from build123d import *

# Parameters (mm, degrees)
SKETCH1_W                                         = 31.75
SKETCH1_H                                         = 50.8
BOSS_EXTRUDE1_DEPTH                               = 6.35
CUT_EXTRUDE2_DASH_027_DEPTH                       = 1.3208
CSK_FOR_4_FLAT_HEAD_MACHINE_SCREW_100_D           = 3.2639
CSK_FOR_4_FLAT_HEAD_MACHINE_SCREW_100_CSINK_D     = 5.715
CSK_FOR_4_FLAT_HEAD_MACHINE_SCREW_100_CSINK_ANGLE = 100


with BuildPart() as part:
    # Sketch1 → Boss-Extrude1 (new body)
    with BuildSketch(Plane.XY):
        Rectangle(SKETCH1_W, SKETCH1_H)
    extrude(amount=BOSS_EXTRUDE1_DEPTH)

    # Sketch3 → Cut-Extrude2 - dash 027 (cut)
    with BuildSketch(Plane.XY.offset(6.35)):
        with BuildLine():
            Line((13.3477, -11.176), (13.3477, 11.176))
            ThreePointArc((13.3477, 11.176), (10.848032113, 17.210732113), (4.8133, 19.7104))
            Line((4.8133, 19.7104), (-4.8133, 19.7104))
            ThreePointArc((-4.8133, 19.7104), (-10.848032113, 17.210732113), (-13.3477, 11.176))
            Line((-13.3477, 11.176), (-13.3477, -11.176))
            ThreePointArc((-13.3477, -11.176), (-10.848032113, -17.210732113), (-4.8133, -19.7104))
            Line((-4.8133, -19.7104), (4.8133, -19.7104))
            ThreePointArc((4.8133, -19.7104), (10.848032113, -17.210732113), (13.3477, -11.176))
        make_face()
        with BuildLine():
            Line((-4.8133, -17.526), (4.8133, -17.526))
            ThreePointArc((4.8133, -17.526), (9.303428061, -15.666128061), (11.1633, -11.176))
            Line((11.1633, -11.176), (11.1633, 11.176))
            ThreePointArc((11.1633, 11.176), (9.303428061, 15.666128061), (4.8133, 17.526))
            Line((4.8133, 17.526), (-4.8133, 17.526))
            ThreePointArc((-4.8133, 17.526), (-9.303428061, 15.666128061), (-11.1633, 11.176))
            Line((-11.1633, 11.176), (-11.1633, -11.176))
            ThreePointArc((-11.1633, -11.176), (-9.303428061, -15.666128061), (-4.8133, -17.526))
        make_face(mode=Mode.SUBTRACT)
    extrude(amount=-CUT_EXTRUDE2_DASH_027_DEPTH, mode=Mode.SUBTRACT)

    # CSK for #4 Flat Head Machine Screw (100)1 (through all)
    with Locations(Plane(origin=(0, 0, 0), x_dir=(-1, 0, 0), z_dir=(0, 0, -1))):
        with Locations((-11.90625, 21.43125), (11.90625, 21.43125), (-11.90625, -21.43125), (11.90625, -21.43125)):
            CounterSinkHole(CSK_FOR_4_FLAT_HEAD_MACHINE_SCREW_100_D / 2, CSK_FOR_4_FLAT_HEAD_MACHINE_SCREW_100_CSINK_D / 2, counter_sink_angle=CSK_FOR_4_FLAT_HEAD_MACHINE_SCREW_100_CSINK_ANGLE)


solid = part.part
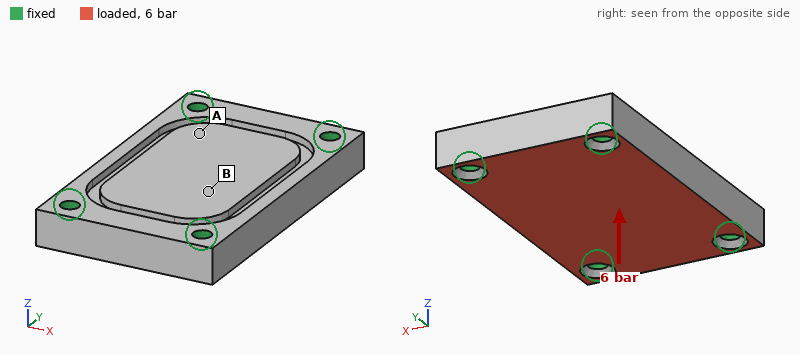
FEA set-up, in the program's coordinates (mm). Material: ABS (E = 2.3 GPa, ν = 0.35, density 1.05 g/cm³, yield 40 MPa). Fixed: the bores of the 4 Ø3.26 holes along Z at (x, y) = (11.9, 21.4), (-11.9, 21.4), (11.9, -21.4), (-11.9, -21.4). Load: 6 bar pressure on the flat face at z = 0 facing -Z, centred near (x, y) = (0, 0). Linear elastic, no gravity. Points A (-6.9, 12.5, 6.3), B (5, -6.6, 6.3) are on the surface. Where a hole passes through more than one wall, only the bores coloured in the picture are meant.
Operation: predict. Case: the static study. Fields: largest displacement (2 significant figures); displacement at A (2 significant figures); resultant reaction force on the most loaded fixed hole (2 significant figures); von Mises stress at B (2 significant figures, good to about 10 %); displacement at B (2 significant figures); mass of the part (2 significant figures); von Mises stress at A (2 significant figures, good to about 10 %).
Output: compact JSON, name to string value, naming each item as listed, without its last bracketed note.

{"largest displacement": "0.20 mm", "displacement at A": "0.12 mm", "resultant reaction force on the most loaded fixed hole": "230 N", "von Mises stress at B": "6.2 MPa", "displacement at B": "0.17 mm", "mass of the part": "10 g", "von Mises stress at A": "3.0 MPa"}
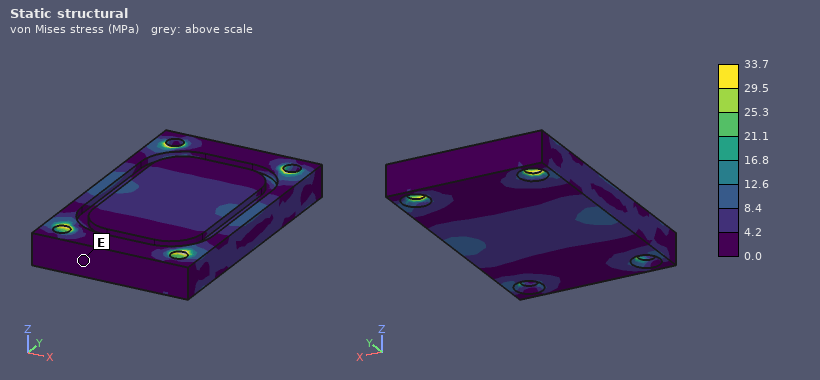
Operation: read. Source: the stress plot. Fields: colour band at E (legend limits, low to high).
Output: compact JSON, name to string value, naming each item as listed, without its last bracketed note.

{"colour band at E": "0.0 to 4.2 MPa"}
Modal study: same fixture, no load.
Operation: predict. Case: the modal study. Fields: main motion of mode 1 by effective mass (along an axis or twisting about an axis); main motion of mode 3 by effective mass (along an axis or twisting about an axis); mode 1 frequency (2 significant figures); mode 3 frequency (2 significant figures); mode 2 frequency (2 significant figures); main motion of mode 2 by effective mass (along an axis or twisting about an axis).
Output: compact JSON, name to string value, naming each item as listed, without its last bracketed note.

{"main motion of mode 1 by effective mass": "along Z", "main motion of mode 3 by effective mass": "along X", "mode 1 frequency": "3900 Hz", "mode 3 frequency": "8500 Hz", "mode 2 frequency": "5700 Hz", "main motion of mode 2 by effective mass": "twisting about Y"}
